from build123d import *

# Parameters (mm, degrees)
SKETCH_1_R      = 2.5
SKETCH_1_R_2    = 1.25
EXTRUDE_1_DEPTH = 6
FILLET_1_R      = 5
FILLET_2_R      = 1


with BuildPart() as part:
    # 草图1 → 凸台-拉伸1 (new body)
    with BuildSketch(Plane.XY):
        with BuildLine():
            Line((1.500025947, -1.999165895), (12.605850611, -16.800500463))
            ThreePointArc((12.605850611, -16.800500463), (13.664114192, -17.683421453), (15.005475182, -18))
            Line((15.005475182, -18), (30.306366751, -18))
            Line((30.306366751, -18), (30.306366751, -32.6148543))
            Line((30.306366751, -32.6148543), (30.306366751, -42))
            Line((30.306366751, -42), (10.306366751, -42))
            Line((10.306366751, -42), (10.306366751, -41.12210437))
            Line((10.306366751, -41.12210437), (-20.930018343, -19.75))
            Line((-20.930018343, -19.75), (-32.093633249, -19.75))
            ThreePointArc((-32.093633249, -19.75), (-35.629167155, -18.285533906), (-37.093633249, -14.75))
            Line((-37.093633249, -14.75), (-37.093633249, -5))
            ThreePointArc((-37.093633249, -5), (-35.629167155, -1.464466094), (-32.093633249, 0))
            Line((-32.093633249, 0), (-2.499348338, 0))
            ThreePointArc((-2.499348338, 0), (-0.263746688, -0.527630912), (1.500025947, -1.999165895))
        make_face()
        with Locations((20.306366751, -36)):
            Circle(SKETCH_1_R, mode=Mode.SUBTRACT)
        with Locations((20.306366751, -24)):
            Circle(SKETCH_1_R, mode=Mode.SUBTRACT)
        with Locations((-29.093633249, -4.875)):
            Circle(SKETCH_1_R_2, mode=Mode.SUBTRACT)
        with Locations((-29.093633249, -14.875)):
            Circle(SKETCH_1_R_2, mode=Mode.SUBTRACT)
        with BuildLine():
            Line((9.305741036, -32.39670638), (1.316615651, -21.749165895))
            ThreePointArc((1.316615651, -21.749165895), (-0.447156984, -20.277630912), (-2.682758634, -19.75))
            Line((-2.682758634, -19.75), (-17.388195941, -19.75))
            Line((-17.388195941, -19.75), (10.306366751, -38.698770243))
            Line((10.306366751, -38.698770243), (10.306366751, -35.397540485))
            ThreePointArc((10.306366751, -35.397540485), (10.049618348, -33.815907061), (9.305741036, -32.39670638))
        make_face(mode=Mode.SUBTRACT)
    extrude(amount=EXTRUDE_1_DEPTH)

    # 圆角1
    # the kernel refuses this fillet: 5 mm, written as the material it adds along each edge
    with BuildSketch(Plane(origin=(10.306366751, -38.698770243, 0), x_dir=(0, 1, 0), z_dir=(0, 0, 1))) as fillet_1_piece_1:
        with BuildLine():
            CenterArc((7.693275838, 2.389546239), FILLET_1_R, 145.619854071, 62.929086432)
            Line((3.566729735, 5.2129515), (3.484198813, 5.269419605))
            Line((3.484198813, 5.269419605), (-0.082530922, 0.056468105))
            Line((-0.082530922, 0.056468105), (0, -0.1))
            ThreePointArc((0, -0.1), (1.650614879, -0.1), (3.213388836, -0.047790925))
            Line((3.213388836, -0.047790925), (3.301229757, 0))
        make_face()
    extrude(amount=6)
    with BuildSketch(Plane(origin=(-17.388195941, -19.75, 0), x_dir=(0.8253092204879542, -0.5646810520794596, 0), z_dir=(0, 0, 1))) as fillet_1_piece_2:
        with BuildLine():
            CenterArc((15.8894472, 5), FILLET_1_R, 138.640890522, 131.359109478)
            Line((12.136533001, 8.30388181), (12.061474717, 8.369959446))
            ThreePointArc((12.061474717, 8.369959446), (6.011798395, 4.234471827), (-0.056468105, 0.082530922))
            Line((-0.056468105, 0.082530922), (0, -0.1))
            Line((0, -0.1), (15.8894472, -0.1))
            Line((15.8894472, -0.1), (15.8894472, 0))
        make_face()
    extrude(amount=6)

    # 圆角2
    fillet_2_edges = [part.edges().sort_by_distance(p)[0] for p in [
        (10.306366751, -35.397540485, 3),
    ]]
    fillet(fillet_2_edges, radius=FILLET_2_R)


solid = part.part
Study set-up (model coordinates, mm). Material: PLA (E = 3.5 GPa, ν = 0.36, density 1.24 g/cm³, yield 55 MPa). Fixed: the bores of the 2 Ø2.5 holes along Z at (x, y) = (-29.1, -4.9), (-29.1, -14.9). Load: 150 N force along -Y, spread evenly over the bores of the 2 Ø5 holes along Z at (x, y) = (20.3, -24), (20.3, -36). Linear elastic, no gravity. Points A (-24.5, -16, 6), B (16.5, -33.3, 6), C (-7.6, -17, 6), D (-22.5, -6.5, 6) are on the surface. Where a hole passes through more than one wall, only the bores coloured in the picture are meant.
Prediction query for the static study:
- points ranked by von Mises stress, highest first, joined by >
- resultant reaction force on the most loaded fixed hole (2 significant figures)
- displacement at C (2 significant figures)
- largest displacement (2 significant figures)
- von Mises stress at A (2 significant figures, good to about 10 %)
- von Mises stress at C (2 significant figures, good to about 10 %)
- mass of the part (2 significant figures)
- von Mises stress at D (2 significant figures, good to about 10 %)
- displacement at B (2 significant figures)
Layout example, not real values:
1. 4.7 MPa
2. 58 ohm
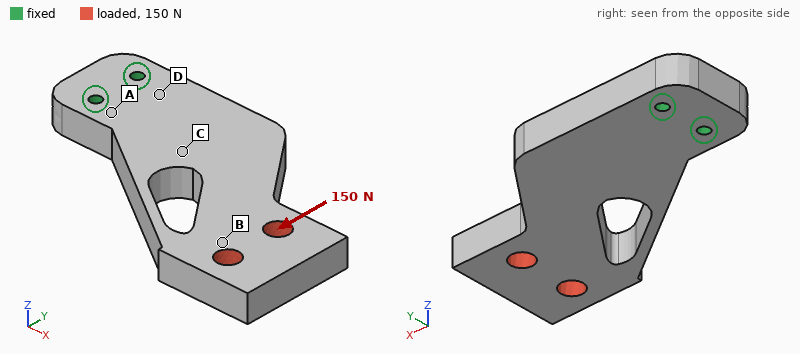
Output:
1. A > D > C > B
2. 660 N
3. 0.17 mm
4. 0.82 mm
5. 13 MPa
6. 4.6 MPa
7. 11 g
8. 9.2 MPa
9. 0.58 mm
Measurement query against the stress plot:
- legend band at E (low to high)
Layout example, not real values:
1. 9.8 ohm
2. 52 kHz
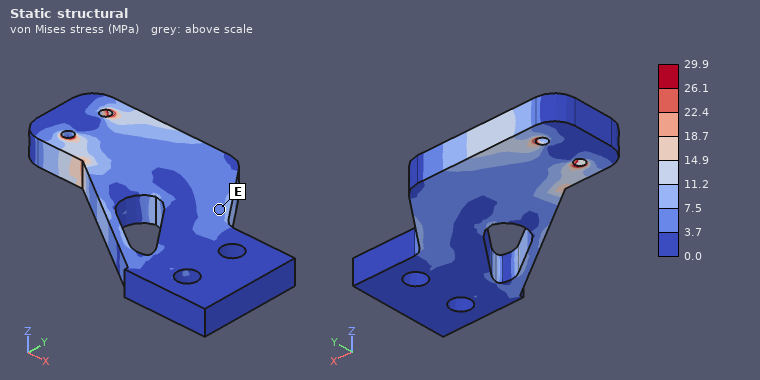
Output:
1. 3.7 to 7.5 MPa
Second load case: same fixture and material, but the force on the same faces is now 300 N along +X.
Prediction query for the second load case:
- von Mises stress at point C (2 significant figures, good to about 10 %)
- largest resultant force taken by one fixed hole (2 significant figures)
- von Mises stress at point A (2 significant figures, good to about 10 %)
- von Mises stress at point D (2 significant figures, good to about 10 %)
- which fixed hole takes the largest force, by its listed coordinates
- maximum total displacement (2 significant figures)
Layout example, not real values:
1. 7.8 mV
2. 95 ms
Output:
1. 8.2 MPa
2. 690 N
3. 15 MPa
4. 5.0 MPa
5. (-29.1, -14.9)
6. 0.82 mm
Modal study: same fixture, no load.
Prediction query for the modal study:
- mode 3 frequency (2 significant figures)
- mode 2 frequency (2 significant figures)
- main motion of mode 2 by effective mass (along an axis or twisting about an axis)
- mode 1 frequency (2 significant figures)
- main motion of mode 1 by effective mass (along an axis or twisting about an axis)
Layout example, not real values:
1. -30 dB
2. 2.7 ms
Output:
1. 1600 Hz
2. 1100 Hz
3. along Y
4. 390 Hz
5. along Z
